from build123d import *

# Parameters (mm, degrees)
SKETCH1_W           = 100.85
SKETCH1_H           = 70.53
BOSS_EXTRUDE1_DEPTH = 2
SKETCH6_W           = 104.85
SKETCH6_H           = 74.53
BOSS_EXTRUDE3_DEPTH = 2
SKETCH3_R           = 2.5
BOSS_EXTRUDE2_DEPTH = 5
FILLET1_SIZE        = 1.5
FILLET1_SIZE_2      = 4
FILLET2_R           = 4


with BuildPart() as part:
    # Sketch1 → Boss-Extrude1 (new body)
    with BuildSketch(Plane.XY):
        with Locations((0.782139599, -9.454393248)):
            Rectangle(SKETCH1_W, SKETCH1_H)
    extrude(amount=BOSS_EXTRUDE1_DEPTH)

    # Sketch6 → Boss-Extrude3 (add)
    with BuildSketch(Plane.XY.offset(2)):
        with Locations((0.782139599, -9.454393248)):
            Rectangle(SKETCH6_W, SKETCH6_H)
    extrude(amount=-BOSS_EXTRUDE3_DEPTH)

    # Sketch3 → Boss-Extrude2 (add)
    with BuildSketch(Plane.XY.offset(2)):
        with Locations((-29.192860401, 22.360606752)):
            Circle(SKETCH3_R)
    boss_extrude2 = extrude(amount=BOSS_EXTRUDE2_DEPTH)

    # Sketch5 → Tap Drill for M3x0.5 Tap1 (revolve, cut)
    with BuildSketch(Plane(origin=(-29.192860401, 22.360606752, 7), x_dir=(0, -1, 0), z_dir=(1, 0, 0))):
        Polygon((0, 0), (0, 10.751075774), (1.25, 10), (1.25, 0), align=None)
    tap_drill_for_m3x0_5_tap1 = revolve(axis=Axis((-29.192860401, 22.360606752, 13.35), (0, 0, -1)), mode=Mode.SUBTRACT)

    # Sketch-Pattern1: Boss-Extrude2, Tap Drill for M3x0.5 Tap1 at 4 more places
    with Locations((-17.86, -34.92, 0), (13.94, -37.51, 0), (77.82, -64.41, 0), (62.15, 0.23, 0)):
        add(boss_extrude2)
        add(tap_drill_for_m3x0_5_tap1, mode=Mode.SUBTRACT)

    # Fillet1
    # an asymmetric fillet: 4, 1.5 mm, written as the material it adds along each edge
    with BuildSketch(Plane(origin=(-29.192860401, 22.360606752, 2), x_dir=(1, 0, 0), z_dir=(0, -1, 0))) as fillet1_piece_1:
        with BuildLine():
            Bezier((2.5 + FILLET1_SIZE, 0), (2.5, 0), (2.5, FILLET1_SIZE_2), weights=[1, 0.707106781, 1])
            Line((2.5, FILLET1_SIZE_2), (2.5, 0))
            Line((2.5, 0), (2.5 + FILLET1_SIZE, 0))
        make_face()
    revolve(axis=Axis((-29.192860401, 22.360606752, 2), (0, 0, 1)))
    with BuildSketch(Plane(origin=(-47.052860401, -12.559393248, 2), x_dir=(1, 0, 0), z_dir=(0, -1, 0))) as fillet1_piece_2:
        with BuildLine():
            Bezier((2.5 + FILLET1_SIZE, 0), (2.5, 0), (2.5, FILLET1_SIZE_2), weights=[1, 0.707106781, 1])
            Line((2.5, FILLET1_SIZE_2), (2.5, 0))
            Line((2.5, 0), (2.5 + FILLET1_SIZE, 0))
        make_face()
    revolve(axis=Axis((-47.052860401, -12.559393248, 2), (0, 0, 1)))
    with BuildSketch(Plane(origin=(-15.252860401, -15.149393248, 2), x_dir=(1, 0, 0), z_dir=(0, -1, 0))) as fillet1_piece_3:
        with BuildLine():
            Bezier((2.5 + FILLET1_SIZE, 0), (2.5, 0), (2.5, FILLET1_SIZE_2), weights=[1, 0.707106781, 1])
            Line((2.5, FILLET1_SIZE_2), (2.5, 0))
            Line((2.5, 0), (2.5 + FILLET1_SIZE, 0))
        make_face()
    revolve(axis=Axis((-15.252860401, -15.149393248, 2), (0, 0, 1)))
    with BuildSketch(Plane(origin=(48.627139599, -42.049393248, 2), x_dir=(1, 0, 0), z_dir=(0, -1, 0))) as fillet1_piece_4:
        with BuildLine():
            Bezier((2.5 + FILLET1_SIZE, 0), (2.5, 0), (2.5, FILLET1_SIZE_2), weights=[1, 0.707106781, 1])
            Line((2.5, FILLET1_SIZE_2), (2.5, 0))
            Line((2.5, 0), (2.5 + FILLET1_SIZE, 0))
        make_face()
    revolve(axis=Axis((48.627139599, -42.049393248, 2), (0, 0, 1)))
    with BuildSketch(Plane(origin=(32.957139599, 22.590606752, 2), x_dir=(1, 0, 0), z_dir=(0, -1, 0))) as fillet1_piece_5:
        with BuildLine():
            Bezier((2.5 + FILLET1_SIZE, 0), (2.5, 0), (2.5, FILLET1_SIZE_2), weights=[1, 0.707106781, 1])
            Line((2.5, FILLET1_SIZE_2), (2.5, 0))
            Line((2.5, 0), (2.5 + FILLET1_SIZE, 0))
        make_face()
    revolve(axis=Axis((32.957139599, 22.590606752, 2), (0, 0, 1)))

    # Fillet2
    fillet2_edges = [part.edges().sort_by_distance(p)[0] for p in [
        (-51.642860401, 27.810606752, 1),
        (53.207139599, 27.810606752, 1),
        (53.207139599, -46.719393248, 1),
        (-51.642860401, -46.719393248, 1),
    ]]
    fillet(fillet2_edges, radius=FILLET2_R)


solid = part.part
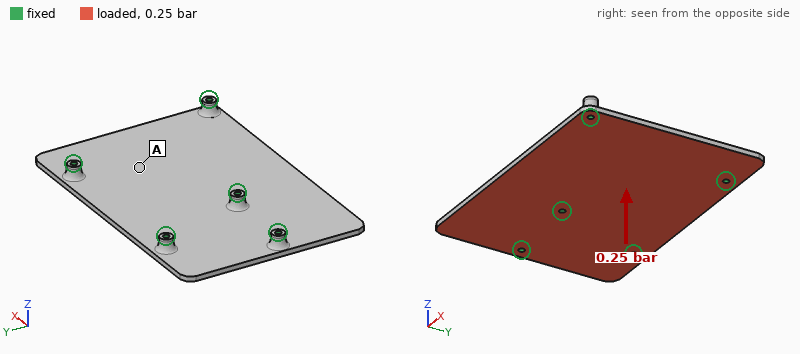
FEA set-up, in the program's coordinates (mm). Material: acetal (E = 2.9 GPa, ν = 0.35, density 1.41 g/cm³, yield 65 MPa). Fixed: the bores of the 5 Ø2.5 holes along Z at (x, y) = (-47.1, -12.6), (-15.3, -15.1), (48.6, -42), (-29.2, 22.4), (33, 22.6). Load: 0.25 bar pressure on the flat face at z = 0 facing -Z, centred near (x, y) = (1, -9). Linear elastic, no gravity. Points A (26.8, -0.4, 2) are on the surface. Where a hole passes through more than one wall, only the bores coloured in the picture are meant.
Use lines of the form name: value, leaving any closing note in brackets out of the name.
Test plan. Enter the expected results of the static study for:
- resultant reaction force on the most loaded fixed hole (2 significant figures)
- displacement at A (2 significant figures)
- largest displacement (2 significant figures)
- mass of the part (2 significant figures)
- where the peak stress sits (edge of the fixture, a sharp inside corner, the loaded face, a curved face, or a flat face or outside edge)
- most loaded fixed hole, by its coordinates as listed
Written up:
resultant reaction force on the most loaded fixed hole: 71 N
displacement at A: 0.56 mm
largest displacement: 1.5 mm
mass of the part: 23 g
where the peak stress sits: a curved face
most loaded fixed hole, by its coordinates as listed: (-15.3, -15.1)
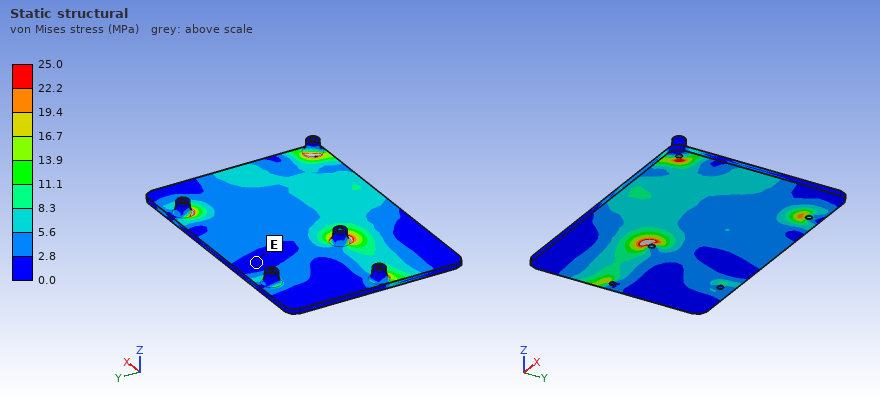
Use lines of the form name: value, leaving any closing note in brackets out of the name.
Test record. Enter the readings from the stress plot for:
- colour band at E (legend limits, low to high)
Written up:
colour band at E: 0.0 to 2.8 MPa
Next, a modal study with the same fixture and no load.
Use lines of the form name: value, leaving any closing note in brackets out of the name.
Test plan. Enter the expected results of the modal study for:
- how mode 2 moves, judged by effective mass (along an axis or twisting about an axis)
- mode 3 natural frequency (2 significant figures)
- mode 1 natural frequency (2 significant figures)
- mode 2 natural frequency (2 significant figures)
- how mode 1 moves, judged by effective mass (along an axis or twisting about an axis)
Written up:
how mode 2 moves, judged by effective mass: along Z
mode 3 natural frequency: 710 Hz
mode 1 natural frequency: 480 Hz
mode 2 natural frequency: 610 Hz
how mode 1 moves, judged by effective mass: along Z
